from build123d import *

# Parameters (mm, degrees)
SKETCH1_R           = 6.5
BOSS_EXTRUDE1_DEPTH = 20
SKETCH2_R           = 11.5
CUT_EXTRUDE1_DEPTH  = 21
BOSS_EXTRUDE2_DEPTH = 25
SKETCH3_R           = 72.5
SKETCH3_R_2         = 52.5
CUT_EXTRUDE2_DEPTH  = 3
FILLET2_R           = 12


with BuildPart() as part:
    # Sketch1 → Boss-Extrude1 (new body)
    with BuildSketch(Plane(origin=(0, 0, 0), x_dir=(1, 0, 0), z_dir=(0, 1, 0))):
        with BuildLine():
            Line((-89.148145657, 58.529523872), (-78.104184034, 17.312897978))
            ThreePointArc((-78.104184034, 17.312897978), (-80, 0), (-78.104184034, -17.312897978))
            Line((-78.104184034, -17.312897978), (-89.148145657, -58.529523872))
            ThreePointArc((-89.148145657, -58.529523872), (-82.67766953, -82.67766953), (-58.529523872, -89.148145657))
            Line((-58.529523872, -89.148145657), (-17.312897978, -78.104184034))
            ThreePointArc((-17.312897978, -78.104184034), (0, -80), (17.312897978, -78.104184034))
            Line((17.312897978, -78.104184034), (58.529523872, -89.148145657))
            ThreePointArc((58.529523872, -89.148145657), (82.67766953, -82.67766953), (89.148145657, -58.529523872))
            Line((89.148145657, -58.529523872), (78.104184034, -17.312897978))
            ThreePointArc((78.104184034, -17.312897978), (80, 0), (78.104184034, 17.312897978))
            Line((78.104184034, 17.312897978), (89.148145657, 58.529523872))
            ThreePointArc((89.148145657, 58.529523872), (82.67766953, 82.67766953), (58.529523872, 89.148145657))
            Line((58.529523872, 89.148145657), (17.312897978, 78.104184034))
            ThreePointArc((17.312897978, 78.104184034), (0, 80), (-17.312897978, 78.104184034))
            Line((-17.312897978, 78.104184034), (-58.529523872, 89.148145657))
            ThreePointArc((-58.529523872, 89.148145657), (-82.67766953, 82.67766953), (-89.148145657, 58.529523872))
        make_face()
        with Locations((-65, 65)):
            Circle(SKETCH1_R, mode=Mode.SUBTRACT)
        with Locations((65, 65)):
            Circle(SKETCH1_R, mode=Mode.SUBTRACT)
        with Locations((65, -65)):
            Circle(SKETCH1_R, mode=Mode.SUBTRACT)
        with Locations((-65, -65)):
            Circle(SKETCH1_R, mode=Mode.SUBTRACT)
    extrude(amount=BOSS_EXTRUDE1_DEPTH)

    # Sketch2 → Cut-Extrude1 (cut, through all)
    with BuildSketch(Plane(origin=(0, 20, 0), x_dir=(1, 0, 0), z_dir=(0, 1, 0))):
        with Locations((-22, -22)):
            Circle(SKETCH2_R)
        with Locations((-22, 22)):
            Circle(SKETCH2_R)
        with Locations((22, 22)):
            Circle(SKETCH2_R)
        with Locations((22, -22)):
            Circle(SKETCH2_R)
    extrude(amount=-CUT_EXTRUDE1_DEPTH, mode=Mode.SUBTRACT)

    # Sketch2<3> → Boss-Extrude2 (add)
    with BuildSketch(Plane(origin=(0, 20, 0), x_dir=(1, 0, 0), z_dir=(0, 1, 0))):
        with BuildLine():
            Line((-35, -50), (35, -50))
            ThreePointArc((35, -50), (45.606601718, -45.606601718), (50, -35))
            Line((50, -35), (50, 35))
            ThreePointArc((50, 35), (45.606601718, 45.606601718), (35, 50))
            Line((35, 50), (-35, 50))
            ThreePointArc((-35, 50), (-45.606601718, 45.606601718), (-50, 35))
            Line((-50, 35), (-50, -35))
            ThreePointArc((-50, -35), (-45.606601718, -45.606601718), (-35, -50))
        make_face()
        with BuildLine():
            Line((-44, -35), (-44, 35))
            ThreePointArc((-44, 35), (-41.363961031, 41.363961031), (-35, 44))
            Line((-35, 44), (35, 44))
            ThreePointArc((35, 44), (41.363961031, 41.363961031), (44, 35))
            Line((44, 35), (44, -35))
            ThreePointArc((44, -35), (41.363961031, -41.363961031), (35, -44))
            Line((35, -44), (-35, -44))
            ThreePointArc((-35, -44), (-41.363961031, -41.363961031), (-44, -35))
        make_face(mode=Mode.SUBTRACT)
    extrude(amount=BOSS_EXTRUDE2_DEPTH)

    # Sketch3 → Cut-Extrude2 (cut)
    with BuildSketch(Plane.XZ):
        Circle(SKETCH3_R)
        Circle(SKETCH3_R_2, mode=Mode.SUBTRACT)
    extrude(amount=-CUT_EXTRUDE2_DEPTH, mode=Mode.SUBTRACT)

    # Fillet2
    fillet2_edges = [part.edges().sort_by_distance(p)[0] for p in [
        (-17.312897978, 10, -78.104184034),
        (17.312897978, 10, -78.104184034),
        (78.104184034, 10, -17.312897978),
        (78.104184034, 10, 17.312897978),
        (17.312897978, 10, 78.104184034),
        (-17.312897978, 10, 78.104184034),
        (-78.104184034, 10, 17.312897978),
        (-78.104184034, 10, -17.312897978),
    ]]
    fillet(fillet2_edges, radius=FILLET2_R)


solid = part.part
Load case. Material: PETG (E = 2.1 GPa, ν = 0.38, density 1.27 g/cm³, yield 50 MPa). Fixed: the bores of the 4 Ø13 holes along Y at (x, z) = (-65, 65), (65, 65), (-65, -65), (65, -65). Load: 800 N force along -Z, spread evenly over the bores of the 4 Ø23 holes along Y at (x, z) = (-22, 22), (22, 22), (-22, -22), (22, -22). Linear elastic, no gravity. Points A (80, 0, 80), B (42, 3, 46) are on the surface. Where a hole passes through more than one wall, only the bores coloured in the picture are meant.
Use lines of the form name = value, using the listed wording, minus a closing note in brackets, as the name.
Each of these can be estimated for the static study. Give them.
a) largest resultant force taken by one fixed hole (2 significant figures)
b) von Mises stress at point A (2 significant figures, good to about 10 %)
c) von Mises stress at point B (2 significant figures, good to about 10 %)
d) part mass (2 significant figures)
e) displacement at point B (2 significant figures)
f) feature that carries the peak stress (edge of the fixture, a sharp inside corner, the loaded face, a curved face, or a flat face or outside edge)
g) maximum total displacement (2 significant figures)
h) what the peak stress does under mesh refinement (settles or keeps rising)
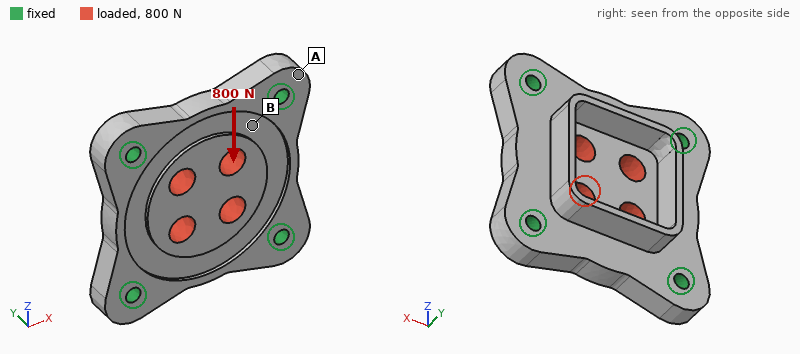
largest resultant force taken by one fixed hole = 220 N
von Mises stress at point A = 0.11 MPa
von Mises stress at point B = 0.32 MPa
part mass = 700 g
displacement at point B = 5.6 µm
feature that carries the peak stress = edge of the fixture
maximum total displacement = 14 µm
what the peak stress does under mesh refinement = keeps rising
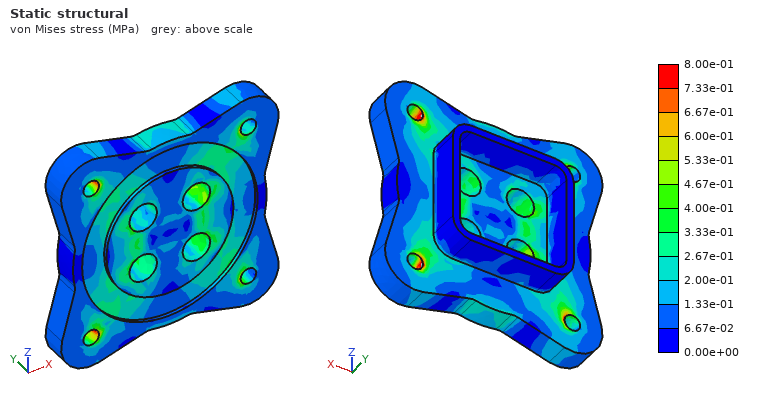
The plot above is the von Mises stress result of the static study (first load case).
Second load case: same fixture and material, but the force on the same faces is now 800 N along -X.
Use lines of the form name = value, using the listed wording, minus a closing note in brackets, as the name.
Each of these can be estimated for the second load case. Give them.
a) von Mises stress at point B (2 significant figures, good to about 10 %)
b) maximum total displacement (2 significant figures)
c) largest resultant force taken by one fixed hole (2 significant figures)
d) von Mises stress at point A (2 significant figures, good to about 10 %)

von Mises stress at point B = 0.32 MPa
maximum total displacement = 14 µm
largest resultant force taken by one fixed hole = 220 N
von Mises stress at point A = 0.11 MPa
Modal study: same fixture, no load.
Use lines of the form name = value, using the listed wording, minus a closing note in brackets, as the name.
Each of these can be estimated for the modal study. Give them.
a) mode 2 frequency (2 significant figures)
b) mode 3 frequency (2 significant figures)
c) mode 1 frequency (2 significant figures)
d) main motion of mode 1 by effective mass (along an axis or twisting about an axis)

mode 2 frequency = 1600 Hz
mode 3 frequency = 1600 Hz
mode 1 frequency = 1000 Hz
main motion of mode 1 by effective mass = along Y
